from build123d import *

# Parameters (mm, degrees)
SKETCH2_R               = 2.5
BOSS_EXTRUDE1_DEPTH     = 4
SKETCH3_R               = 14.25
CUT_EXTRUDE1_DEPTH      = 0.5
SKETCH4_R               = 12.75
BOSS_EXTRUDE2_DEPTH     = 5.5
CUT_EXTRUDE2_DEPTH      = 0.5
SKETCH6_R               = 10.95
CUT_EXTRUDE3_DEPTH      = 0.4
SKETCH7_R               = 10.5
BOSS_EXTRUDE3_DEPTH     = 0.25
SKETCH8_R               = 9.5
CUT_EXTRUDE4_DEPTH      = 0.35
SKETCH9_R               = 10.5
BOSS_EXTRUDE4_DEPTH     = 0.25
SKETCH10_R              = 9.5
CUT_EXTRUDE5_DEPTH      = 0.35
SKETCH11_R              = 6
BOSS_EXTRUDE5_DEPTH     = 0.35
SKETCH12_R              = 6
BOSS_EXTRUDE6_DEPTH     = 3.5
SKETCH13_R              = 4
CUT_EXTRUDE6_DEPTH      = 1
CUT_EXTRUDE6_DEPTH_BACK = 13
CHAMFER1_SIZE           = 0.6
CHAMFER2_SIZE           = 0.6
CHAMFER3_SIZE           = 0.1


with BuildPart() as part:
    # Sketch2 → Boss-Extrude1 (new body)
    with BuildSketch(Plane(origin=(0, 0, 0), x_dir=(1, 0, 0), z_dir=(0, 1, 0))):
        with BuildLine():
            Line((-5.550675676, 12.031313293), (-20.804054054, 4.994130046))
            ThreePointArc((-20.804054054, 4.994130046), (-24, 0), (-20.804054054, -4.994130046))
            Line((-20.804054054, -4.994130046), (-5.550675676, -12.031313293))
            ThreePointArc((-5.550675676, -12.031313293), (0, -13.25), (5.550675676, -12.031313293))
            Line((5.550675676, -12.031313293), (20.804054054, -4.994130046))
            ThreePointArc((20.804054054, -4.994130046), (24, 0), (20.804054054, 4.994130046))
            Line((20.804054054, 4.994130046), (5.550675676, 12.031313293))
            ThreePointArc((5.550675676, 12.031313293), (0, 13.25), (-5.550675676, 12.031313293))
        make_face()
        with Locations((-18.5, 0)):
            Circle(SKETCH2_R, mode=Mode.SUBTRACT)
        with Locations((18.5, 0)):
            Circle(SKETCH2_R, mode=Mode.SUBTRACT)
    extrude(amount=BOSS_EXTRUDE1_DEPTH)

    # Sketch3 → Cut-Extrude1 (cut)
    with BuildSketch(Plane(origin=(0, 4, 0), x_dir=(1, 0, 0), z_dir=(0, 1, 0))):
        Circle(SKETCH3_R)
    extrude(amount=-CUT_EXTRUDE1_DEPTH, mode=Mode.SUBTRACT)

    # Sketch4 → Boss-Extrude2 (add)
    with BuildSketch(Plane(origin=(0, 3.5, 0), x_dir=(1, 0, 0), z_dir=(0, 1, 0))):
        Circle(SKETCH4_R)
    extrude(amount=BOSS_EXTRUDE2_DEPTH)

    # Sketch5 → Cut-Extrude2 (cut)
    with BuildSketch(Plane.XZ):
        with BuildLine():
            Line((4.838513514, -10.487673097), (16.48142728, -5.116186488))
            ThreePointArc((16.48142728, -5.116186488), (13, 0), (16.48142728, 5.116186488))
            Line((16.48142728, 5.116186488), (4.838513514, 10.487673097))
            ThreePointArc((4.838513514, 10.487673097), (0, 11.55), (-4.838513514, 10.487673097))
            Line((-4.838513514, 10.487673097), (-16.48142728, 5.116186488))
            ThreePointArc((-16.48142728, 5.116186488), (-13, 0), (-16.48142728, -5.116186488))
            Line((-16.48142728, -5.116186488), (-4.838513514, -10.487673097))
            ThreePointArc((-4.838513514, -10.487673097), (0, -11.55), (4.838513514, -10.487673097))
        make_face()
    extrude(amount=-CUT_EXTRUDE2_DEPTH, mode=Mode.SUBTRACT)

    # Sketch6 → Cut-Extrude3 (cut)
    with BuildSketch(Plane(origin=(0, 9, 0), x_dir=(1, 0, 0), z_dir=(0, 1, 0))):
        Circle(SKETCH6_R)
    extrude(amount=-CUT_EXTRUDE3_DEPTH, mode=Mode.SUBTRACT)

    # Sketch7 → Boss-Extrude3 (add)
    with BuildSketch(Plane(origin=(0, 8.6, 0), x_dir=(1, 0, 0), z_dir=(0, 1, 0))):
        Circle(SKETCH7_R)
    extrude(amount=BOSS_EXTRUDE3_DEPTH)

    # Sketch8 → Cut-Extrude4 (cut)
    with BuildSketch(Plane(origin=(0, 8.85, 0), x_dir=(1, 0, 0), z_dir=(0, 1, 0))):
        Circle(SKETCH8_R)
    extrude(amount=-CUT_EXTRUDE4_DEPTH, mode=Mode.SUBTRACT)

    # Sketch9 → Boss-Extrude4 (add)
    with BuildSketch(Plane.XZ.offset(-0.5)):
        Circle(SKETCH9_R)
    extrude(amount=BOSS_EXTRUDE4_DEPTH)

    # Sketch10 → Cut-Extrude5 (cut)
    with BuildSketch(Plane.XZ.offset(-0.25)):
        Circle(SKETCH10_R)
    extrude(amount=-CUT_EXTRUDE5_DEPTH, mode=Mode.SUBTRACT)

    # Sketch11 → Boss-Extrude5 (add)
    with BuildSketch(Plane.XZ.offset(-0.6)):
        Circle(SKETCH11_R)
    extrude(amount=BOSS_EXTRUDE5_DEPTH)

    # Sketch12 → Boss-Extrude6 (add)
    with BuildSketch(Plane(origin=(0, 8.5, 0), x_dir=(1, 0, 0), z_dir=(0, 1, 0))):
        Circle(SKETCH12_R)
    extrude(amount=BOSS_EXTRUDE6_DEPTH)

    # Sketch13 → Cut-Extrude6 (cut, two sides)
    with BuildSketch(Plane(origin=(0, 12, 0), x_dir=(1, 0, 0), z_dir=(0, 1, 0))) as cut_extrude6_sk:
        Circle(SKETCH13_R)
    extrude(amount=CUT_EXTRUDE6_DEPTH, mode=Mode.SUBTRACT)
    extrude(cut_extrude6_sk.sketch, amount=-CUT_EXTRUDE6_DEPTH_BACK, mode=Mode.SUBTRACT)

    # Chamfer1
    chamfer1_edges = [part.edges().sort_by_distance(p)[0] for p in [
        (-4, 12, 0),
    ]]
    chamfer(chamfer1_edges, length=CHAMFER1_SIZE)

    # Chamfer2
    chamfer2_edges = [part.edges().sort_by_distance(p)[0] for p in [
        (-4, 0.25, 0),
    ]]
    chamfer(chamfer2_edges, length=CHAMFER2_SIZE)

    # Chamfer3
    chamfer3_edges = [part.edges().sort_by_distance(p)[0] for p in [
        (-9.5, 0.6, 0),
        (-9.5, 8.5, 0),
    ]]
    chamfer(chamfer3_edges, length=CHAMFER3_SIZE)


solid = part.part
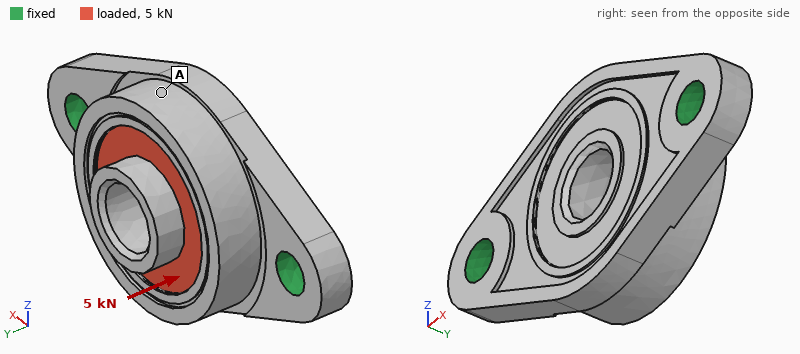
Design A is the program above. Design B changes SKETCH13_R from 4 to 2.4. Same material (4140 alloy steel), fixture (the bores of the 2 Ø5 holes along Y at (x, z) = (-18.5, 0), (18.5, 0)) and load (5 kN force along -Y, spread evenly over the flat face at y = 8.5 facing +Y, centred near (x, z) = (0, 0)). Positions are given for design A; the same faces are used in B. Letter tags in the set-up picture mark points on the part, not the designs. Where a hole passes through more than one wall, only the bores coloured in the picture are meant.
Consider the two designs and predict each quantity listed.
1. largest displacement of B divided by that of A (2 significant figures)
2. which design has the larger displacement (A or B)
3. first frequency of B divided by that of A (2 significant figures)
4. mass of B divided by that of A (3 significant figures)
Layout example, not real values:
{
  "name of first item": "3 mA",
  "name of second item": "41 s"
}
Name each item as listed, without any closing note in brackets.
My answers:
{
  "largest displacement of B divided by that of A": "0.90",
  "which design has the larger displacement": "A",
  "first frequency of B divided by that of A": "0.98",
  "mass of B divided by that of A": "1.07"
}
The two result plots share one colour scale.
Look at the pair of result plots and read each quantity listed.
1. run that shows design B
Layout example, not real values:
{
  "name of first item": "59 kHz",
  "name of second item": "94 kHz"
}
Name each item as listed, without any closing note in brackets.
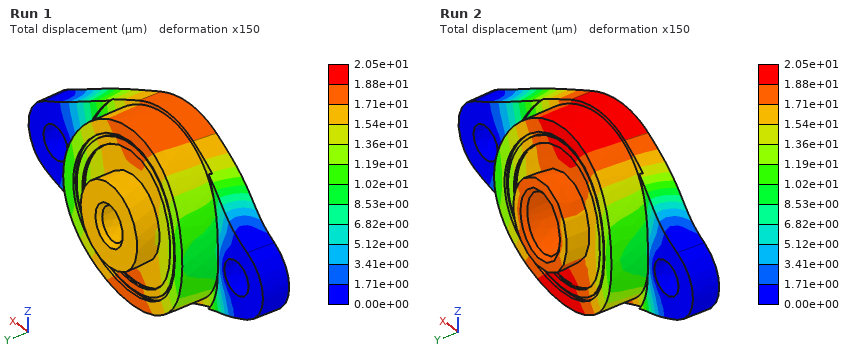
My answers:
{
  "run that shows design B": "Run 1"
}
